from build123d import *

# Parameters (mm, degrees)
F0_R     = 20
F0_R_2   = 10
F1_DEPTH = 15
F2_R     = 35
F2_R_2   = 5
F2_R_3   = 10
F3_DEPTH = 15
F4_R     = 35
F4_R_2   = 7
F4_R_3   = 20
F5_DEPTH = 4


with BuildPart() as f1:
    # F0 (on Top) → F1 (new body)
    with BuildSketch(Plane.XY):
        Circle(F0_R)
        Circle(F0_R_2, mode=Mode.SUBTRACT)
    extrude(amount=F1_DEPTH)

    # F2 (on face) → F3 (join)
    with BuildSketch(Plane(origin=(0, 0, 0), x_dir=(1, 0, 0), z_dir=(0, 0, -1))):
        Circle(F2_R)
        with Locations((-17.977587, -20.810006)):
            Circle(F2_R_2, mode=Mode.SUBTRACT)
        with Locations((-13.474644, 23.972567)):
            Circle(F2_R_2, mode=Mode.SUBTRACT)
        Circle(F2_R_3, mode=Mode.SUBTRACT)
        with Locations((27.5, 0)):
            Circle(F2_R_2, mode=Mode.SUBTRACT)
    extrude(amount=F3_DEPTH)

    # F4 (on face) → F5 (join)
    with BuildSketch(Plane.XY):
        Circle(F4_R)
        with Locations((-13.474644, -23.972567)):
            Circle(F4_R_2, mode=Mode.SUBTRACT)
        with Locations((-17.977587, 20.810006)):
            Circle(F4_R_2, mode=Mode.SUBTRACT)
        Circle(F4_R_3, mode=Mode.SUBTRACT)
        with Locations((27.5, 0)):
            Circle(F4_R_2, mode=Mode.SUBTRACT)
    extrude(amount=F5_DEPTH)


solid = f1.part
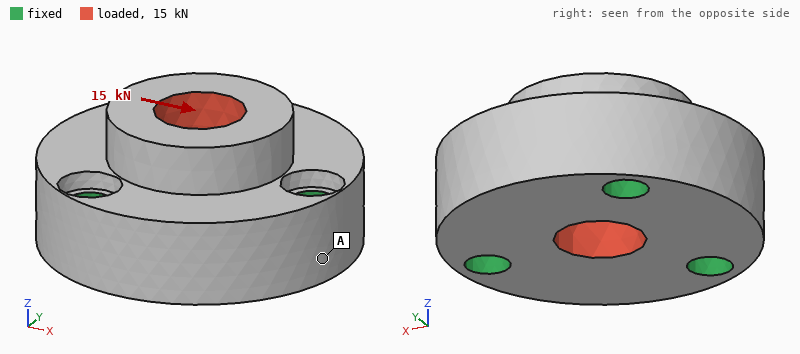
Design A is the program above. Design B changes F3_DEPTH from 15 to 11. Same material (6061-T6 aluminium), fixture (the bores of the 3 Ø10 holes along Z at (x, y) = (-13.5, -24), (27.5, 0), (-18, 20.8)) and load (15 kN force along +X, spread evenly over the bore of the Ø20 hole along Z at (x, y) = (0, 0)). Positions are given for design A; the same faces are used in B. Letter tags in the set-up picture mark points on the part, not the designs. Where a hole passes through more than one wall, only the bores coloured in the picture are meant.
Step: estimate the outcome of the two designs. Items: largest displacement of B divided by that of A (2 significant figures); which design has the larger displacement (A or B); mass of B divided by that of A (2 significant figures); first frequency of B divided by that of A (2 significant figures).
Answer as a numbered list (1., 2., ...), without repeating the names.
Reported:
1. 1.2
2. B
3. 0.82
4. 0.89
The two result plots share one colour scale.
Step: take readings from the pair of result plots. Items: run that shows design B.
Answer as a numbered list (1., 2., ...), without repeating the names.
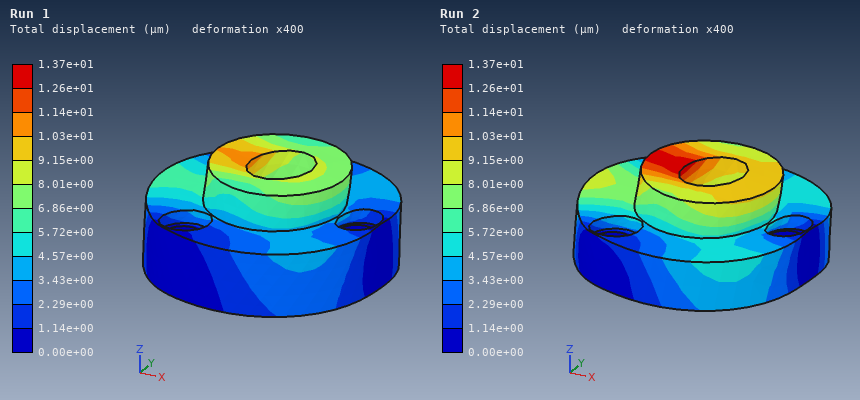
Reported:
1. Run 2
